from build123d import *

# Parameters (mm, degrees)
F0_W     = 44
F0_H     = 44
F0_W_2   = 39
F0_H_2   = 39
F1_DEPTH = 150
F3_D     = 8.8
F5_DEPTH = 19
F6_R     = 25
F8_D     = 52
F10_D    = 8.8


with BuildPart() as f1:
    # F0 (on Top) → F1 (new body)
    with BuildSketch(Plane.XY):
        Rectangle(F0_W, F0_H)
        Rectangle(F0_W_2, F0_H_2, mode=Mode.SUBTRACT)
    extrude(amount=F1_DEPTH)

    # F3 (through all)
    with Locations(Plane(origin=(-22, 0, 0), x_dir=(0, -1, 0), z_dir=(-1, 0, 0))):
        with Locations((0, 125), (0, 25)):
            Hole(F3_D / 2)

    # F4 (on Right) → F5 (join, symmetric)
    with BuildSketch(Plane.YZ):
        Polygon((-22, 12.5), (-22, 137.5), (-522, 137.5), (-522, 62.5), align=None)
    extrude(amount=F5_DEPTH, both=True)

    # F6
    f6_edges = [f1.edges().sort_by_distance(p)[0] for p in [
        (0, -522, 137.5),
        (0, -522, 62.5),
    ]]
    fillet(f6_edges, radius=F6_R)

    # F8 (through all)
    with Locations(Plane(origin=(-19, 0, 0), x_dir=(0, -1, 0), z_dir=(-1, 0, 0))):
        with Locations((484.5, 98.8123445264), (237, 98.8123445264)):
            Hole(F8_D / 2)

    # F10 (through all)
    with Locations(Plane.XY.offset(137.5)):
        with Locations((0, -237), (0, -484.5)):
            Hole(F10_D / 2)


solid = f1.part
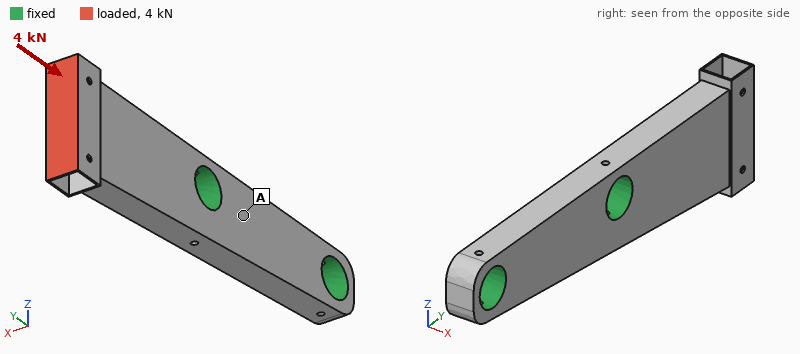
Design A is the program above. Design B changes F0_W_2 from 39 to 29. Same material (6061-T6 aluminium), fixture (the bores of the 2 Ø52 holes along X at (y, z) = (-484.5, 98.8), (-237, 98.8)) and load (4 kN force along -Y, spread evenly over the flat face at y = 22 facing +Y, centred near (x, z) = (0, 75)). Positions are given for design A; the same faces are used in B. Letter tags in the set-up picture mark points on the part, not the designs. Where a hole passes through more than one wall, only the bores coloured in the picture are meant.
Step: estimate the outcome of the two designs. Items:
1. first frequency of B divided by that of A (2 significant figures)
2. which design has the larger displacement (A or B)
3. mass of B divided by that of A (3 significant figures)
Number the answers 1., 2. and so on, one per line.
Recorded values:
1. 0.92
2. A
3. 1.03
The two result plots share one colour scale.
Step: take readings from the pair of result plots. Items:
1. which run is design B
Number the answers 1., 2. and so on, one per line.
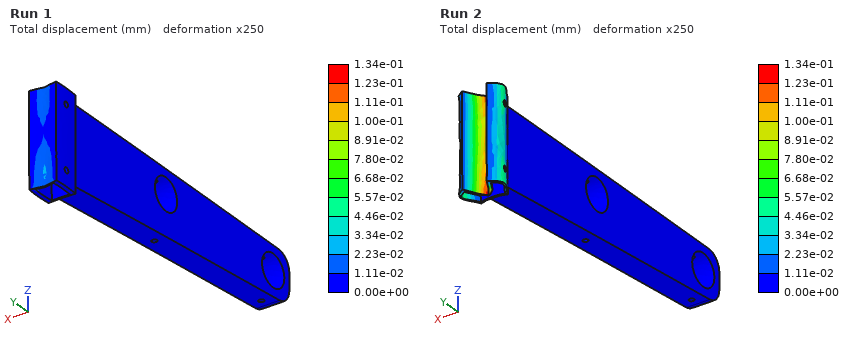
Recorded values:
1. Run 1
